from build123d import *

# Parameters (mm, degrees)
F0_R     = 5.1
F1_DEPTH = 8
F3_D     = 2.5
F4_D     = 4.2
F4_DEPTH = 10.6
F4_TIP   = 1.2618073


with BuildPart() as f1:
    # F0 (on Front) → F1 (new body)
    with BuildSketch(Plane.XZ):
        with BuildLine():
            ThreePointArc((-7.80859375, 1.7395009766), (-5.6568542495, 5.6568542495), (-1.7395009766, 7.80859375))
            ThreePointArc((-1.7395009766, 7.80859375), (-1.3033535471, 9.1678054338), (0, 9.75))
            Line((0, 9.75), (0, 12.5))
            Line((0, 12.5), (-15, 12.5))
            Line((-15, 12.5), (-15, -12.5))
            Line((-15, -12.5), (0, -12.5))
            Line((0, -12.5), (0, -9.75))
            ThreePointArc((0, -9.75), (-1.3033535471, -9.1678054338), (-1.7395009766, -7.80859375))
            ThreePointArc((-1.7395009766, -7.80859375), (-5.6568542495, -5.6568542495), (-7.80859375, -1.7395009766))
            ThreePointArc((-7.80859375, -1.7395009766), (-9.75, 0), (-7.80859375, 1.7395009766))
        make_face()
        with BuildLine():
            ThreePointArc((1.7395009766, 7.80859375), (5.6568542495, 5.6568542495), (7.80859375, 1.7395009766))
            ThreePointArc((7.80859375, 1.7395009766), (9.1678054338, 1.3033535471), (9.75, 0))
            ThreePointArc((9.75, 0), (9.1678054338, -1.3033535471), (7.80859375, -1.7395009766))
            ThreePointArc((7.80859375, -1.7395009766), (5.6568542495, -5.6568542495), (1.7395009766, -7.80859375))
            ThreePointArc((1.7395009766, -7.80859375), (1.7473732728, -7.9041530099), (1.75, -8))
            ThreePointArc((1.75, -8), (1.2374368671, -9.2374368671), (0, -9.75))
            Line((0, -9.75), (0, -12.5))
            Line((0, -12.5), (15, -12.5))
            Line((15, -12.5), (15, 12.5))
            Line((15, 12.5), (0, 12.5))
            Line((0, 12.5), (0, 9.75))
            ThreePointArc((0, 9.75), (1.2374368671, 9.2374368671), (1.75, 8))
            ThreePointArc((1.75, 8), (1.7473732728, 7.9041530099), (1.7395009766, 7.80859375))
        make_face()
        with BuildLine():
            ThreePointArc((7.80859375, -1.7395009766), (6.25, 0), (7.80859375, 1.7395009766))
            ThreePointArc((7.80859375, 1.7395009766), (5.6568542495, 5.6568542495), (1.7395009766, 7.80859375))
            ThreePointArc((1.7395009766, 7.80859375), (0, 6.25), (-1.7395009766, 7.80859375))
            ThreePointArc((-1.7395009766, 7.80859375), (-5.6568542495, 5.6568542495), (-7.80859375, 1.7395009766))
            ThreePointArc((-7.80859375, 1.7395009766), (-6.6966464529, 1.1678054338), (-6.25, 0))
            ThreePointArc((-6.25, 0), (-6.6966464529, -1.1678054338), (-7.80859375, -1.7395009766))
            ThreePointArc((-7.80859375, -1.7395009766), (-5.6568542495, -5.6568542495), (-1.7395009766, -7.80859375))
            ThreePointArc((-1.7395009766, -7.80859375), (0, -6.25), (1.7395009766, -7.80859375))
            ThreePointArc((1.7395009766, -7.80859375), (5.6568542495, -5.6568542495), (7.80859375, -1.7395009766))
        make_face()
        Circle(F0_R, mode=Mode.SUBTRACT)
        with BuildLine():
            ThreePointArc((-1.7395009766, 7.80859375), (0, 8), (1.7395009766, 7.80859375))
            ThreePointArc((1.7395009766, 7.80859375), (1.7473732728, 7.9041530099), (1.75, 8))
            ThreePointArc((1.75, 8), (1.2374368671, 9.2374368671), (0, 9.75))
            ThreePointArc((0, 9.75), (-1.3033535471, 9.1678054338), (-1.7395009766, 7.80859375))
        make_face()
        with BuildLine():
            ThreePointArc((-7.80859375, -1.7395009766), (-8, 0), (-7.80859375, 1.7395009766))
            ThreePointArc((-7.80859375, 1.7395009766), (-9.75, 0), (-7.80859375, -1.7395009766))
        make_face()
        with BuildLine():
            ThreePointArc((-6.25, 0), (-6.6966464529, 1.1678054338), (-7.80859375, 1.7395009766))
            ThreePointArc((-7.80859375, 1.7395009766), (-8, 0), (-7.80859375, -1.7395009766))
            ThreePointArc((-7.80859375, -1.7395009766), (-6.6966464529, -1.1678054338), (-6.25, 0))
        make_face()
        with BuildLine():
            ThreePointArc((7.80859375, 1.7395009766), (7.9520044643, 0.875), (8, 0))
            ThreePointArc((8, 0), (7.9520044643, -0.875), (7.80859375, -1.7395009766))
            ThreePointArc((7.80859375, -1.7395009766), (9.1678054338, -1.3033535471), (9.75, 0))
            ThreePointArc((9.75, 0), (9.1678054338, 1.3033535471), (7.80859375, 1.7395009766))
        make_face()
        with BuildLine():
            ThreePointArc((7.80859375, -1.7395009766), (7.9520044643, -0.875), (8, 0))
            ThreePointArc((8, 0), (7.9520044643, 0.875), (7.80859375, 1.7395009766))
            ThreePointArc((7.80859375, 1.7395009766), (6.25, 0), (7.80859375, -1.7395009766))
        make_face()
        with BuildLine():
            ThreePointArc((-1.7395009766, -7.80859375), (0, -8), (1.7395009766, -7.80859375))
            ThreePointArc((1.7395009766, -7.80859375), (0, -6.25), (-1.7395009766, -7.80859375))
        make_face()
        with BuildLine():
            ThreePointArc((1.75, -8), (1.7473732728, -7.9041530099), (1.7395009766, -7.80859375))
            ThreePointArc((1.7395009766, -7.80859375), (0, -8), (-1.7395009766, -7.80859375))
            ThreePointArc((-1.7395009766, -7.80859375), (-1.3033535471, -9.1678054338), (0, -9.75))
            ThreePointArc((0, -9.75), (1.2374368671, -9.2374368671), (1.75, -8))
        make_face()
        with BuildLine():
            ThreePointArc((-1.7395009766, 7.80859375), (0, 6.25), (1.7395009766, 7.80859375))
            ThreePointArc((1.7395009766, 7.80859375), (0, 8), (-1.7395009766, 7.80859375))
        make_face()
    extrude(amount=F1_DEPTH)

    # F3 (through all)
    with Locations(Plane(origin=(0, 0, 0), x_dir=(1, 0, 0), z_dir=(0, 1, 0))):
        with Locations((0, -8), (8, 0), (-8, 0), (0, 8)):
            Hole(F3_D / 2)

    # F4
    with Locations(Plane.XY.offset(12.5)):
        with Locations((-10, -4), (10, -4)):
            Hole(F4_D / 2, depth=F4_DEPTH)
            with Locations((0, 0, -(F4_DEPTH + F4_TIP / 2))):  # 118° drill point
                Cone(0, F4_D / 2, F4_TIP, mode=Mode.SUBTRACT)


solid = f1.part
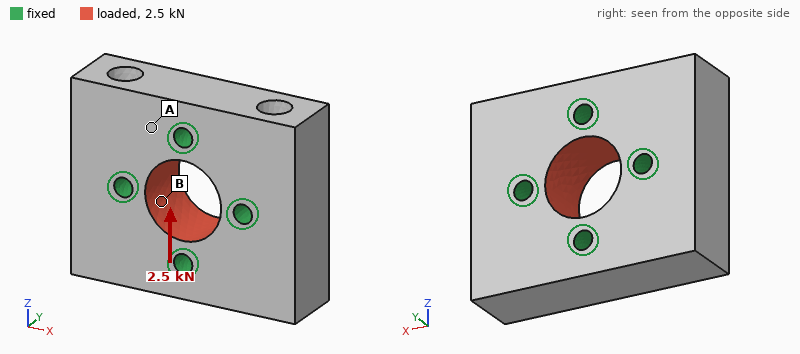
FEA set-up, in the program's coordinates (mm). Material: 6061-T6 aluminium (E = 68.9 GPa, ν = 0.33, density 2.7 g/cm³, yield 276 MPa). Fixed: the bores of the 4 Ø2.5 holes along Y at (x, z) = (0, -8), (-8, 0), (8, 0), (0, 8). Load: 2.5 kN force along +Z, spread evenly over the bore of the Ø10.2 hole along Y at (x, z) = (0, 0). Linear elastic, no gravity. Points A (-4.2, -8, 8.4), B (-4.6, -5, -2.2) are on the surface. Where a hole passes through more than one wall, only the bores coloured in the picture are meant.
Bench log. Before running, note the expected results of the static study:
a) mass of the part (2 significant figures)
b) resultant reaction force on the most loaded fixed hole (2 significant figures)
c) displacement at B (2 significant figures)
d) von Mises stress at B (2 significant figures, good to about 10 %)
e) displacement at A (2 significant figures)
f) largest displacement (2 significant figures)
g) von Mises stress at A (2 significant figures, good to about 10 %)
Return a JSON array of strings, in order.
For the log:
["13 g", "640 N", "0.91 µm", "15 MPa", "0.47 µm", "1.0 µm", "4.9 MPa"]
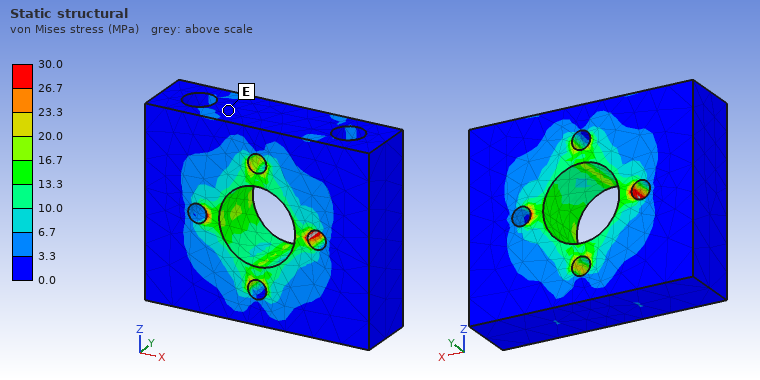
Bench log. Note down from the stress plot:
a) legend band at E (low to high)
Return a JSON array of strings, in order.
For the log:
["0.0 to 3.3 MPa"]
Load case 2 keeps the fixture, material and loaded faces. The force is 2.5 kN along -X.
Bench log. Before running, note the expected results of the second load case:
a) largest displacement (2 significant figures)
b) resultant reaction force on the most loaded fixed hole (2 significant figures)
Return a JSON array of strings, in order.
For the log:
["1.0 µm", "630 N"]
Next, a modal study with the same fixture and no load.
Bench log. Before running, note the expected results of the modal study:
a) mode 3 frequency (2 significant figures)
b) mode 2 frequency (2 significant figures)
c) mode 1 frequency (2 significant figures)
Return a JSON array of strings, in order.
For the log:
["41 kHz", "40 kHz", "39 kHz"]
